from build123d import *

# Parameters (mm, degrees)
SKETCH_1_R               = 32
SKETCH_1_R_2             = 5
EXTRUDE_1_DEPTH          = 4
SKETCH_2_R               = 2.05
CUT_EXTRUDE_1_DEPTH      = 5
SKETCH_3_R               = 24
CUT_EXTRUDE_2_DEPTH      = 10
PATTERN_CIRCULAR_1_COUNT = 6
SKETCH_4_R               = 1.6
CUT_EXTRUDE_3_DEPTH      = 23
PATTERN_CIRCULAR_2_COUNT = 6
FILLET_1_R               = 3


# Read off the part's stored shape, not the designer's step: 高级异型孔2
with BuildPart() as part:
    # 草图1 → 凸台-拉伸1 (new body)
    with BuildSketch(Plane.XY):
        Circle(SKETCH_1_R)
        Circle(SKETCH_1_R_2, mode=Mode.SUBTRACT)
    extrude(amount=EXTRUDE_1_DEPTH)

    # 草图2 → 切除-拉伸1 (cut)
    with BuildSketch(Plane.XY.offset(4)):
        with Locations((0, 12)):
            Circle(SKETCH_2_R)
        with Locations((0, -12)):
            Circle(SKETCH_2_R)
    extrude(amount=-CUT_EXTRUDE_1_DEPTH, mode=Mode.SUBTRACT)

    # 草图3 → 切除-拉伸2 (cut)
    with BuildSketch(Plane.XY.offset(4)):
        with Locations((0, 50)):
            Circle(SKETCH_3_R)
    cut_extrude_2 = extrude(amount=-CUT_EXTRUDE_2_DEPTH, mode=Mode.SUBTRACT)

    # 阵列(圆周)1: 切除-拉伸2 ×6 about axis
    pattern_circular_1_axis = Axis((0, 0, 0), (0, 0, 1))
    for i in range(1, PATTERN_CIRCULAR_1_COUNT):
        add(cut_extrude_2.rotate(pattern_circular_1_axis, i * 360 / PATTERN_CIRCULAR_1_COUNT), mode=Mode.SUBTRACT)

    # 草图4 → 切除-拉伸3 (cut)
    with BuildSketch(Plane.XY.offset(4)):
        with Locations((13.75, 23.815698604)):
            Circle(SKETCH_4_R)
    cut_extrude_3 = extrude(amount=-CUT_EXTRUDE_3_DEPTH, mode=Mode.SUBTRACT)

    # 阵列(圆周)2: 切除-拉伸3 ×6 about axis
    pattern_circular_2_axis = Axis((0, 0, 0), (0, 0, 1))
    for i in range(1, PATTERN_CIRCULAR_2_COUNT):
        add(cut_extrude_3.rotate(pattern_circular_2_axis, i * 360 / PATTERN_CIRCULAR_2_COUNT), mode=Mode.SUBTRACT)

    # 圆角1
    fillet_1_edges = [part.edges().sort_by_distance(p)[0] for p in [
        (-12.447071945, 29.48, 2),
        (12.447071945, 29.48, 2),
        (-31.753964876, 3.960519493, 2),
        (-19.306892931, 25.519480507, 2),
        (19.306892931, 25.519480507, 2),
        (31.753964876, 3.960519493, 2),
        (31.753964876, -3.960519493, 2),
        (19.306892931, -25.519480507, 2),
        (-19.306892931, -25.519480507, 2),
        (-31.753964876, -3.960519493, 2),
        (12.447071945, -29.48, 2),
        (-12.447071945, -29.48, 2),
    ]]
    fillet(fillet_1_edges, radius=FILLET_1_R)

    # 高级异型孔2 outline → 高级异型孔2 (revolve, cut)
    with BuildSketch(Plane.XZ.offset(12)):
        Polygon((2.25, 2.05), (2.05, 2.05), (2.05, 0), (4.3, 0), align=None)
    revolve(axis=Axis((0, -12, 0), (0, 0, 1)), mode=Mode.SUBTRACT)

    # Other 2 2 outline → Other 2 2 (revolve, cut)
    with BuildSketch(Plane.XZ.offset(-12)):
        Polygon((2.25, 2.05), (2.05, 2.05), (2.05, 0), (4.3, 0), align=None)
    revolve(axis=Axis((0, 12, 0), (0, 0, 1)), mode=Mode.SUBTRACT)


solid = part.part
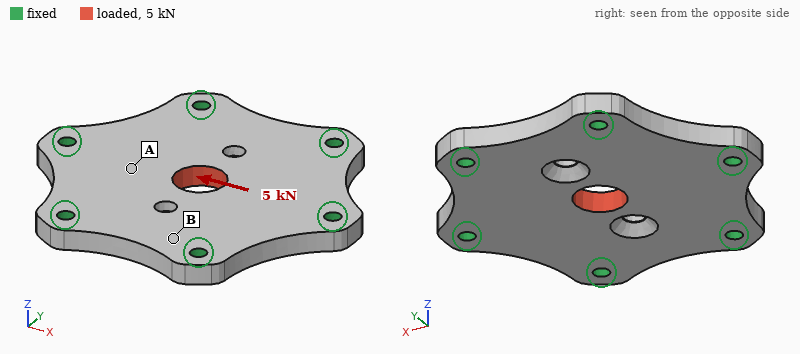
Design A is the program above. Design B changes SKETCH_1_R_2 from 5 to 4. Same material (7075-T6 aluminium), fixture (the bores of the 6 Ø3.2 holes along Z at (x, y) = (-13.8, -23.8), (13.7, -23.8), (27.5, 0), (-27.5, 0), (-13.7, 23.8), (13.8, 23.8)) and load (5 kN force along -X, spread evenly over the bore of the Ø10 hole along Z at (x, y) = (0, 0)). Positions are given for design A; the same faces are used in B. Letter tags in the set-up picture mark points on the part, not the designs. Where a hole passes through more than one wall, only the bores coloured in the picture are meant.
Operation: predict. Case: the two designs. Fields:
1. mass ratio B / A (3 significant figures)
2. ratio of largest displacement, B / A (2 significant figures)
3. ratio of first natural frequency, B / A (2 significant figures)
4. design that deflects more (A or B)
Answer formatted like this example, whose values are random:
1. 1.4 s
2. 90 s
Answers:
1. 1.01
2. 1.1
3. 0.99
4. B
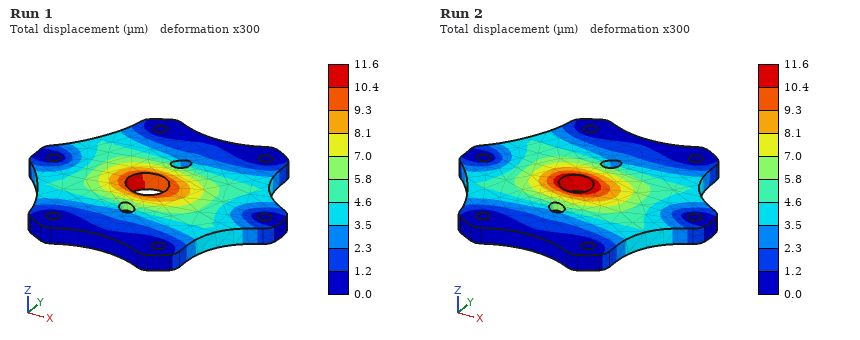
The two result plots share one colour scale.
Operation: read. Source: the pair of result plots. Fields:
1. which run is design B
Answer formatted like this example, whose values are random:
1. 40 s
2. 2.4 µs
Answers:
1. Run 2
